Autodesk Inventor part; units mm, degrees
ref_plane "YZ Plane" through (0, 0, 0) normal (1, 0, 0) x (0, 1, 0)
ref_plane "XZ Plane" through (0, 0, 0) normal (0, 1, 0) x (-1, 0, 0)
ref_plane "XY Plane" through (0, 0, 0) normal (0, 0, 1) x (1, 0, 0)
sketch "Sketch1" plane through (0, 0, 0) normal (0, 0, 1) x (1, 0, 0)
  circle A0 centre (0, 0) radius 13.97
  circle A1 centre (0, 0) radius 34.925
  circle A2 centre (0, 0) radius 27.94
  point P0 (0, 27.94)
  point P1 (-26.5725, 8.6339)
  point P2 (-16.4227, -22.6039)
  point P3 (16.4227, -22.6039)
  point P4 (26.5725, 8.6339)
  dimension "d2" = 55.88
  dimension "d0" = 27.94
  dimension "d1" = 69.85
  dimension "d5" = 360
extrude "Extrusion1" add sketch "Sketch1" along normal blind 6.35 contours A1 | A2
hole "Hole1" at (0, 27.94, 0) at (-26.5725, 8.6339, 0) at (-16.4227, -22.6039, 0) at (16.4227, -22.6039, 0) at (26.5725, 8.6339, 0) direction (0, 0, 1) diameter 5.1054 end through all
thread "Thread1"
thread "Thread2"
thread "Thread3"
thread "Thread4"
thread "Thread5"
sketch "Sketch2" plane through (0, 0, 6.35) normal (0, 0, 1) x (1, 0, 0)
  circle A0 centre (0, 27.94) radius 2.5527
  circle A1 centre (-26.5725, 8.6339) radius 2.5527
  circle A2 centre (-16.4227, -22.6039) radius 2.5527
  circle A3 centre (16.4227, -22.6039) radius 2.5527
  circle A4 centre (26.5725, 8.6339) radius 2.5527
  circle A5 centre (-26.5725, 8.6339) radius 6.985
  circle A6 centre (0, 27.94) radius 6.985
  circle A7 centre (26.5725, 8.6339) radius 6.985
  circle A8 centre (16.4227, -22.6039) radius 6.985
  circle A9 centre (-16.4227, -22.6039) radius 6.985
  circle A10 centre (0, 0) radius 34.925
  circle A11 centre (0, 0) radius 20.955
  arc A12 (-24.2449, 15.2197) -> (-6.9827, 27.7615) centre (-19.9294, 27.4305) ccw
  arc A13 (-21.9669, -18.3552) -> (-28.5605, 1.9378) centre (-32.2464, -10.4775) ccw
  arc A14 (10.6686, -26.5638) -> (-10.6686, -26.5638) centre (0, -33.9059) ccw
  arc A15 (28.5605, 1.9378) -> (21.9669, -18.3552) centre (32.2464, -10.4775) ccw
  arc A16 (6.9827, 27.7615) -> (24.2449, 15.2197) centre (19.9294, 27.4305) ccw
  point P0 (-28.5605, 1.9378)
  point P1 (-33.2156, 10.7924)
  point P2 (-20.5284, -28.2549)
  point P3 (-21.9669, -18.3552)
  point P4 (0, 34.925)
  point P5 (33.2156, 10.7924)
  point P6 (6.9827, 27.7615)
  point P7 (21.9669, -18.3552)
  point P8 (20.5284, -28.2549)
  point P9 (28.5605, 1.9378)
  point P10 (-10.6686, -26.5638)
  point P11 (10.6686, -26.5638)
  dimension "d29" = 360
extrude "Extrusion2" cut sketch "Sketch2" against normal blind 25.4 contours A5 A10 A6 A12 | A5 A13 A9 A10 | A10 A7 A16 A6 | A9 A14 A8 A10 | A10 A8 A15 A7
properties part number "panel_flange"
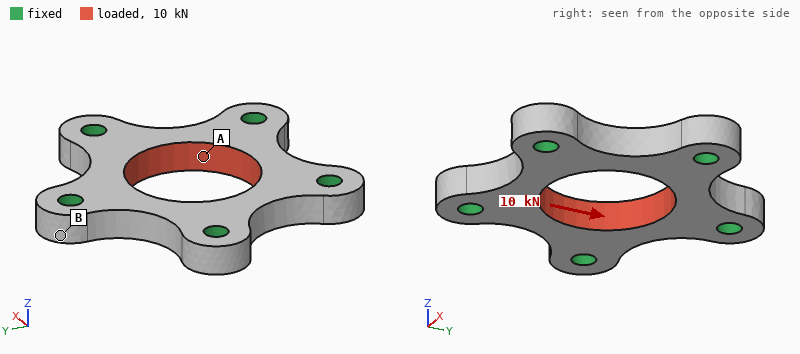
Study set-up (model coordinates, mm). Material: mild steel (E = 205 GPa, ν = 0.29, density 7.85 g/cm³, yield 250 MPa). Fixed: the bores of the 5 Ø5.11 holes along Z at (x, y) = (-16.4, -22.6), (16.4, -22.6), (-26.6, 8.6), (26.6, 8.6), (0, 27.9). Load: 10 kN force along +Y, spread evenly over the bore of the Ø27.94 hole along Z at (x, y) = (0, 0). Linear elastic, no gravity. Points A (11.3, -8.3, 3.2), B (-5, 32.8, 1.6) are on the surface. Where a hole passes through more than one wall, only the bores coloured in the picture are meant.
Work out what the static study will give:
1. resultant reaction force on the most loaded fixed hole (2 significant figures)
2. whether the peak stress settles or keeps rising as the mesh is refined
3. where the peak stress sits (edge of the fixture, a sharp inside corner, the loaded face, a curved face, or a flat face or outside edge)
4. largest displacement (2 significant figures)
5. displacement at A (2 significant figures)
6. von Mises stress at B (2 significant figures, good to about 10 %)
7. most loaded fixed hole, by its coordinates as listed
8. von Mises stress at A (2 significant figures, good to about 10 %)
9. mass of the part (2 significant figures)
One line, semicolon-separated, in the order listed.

3.1 kN; keeps rising; edge of the fixture; 3.7 µm; 1.9 µm; 10 MPa; (0, 27.9); 37 MPa; 82 g
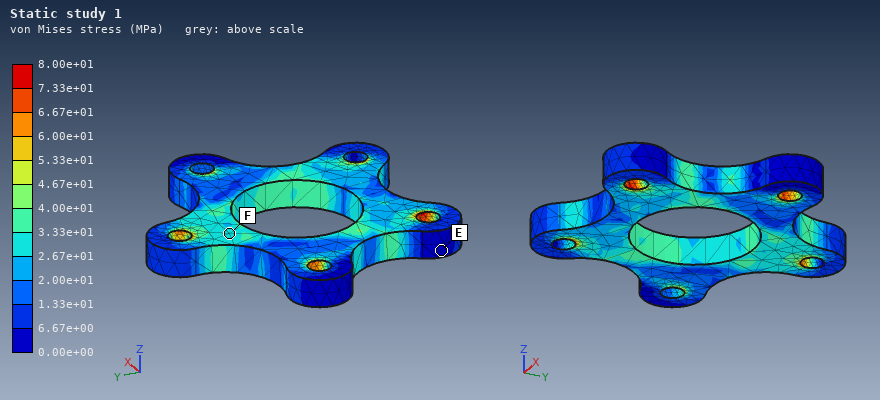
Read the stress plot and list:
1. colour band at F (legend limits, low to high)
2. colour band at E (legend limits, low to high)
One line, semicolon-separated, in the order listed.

2.67e+01 to 3.33e+01 MPa; 0.00e+00 to 6.67e+00 MPa
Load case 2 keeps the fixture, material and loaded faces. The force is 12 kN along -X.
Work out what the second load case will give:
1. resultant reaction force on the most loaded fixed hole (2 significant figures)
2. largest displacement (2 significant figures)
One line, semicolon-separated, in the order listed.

3.5 kN; 4.4 µm
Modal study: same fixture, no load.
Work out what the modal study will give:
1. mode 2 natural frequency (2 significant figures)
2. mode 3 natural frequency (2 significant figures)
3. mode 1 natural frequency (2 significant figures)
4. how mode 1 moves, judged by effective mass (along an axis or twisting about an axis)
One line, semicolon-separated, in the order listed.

27 kHz; 27 kHz; 23 kHz; along Z
